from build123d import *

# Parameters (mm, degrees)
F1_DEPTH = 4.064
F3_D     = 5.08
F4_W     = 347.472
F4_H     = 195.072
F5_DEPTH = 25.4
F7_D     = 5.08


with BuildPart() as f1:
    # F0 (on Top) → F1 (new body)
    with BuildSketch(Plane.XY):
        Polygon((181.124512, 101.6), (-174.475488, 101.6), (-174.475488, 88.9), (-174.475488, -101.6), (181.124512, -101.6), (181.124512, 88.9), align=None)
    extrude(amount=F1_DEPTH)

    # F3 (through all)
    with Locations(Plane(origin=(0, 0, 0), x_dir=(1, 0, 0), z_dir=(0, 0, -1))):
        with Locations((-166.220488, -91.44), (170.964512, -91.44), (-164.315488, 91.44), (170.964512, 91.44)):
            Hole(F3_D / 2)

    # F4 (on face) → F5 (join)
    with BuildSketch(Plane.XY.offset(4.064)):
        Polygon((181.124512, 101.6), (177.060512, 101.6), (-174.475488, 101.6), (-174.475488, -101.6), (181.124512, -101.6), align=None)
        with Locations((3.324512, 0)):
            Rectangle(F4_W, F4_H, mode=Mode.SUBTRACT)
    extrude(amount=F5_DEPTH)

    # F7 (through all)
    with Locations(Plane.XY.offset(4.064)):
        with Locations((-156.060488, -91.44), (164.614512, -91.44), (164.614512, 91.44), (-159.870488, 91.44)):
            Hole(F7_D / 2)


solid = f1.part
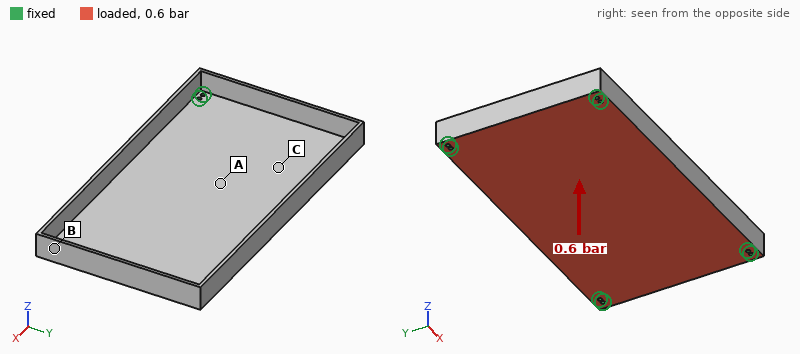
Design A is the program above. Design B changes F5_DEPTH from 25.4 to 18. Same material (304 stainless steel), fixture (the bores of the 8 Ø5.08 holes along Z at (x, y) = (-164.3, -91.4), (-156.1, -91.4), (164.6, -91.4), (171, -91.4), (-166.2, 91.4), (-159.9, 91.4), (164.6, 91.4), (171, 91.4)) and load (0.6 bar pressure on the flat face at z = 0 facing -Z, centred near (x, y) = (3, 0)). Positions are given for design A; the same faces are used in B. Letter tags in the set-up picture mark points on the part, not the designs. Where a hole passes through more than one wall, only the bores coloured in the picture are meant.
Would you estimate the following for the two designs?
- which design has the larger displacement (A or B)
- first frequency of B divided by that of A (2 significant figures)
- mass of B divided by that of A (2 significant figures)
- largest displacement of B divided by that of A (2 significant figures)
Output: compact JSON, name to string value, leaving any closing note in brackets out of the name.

{"which design has the larger displacement": "B", "first frequency of B divided by that of A": "0.93", "mass of B divided by that of A": "0.92", "largest displacement of B divided by that of A": "1.1"}
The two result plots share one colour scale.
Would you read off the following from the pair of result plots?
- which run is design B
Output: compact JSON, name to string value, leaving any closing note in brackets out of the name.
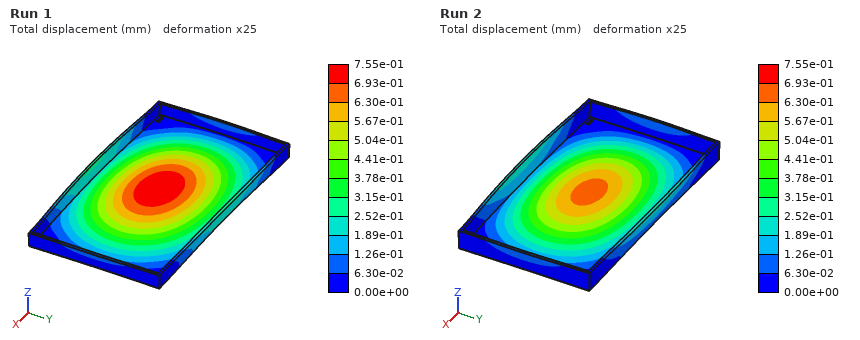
{"which run is design B": "Run 1"}
